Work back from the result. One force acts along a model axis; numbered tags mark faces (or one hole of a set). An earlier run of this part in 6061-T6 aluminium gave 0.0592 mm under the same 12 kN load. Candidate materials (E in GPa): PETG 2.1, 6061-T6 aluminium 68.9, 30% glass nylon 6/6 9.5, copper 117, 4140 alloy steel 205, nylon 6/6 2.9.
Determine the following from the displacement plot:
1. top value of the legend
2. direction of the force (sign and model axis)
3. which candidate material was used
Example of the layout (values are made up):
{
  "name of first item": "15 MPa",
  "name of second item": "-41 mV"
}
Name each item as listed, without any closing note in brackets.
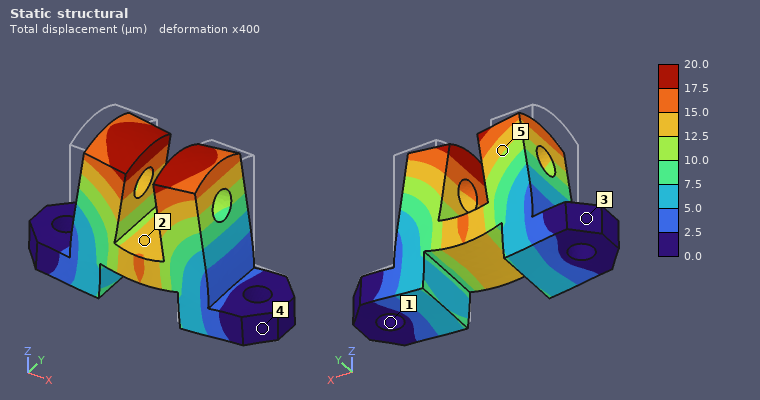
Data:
{
  "top value of the legend": "20.0 µm",
  "direction of the force": "-Z",
  "which candidate material was used": "4140 alloy steel"
}
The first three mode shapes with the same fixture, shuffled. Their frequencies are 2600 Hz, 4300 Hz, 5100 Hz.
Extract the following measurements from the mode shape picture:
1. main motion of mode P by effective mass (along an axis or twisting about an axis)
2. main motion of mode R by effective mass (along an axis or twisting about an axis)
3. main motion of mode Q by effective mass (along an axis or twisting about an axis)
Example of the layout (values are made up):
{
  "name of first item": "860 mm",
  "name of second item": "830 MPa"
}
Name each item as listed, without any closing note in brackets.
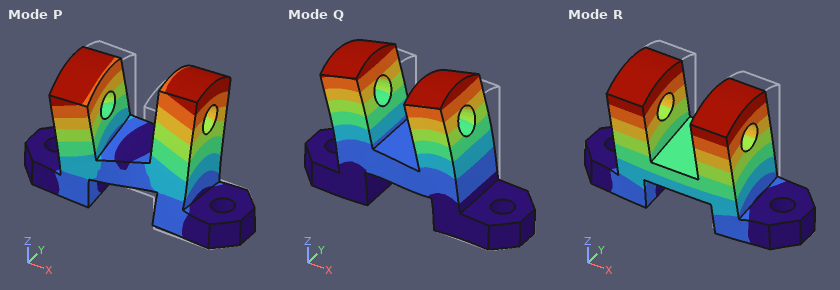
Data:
{
  "main motion of mode P by effective mass": "twisting about Z",
  "main motion of mode R by effective mass": "along Y",
  "main motion of mode Q by effective mass": "along X"
}
